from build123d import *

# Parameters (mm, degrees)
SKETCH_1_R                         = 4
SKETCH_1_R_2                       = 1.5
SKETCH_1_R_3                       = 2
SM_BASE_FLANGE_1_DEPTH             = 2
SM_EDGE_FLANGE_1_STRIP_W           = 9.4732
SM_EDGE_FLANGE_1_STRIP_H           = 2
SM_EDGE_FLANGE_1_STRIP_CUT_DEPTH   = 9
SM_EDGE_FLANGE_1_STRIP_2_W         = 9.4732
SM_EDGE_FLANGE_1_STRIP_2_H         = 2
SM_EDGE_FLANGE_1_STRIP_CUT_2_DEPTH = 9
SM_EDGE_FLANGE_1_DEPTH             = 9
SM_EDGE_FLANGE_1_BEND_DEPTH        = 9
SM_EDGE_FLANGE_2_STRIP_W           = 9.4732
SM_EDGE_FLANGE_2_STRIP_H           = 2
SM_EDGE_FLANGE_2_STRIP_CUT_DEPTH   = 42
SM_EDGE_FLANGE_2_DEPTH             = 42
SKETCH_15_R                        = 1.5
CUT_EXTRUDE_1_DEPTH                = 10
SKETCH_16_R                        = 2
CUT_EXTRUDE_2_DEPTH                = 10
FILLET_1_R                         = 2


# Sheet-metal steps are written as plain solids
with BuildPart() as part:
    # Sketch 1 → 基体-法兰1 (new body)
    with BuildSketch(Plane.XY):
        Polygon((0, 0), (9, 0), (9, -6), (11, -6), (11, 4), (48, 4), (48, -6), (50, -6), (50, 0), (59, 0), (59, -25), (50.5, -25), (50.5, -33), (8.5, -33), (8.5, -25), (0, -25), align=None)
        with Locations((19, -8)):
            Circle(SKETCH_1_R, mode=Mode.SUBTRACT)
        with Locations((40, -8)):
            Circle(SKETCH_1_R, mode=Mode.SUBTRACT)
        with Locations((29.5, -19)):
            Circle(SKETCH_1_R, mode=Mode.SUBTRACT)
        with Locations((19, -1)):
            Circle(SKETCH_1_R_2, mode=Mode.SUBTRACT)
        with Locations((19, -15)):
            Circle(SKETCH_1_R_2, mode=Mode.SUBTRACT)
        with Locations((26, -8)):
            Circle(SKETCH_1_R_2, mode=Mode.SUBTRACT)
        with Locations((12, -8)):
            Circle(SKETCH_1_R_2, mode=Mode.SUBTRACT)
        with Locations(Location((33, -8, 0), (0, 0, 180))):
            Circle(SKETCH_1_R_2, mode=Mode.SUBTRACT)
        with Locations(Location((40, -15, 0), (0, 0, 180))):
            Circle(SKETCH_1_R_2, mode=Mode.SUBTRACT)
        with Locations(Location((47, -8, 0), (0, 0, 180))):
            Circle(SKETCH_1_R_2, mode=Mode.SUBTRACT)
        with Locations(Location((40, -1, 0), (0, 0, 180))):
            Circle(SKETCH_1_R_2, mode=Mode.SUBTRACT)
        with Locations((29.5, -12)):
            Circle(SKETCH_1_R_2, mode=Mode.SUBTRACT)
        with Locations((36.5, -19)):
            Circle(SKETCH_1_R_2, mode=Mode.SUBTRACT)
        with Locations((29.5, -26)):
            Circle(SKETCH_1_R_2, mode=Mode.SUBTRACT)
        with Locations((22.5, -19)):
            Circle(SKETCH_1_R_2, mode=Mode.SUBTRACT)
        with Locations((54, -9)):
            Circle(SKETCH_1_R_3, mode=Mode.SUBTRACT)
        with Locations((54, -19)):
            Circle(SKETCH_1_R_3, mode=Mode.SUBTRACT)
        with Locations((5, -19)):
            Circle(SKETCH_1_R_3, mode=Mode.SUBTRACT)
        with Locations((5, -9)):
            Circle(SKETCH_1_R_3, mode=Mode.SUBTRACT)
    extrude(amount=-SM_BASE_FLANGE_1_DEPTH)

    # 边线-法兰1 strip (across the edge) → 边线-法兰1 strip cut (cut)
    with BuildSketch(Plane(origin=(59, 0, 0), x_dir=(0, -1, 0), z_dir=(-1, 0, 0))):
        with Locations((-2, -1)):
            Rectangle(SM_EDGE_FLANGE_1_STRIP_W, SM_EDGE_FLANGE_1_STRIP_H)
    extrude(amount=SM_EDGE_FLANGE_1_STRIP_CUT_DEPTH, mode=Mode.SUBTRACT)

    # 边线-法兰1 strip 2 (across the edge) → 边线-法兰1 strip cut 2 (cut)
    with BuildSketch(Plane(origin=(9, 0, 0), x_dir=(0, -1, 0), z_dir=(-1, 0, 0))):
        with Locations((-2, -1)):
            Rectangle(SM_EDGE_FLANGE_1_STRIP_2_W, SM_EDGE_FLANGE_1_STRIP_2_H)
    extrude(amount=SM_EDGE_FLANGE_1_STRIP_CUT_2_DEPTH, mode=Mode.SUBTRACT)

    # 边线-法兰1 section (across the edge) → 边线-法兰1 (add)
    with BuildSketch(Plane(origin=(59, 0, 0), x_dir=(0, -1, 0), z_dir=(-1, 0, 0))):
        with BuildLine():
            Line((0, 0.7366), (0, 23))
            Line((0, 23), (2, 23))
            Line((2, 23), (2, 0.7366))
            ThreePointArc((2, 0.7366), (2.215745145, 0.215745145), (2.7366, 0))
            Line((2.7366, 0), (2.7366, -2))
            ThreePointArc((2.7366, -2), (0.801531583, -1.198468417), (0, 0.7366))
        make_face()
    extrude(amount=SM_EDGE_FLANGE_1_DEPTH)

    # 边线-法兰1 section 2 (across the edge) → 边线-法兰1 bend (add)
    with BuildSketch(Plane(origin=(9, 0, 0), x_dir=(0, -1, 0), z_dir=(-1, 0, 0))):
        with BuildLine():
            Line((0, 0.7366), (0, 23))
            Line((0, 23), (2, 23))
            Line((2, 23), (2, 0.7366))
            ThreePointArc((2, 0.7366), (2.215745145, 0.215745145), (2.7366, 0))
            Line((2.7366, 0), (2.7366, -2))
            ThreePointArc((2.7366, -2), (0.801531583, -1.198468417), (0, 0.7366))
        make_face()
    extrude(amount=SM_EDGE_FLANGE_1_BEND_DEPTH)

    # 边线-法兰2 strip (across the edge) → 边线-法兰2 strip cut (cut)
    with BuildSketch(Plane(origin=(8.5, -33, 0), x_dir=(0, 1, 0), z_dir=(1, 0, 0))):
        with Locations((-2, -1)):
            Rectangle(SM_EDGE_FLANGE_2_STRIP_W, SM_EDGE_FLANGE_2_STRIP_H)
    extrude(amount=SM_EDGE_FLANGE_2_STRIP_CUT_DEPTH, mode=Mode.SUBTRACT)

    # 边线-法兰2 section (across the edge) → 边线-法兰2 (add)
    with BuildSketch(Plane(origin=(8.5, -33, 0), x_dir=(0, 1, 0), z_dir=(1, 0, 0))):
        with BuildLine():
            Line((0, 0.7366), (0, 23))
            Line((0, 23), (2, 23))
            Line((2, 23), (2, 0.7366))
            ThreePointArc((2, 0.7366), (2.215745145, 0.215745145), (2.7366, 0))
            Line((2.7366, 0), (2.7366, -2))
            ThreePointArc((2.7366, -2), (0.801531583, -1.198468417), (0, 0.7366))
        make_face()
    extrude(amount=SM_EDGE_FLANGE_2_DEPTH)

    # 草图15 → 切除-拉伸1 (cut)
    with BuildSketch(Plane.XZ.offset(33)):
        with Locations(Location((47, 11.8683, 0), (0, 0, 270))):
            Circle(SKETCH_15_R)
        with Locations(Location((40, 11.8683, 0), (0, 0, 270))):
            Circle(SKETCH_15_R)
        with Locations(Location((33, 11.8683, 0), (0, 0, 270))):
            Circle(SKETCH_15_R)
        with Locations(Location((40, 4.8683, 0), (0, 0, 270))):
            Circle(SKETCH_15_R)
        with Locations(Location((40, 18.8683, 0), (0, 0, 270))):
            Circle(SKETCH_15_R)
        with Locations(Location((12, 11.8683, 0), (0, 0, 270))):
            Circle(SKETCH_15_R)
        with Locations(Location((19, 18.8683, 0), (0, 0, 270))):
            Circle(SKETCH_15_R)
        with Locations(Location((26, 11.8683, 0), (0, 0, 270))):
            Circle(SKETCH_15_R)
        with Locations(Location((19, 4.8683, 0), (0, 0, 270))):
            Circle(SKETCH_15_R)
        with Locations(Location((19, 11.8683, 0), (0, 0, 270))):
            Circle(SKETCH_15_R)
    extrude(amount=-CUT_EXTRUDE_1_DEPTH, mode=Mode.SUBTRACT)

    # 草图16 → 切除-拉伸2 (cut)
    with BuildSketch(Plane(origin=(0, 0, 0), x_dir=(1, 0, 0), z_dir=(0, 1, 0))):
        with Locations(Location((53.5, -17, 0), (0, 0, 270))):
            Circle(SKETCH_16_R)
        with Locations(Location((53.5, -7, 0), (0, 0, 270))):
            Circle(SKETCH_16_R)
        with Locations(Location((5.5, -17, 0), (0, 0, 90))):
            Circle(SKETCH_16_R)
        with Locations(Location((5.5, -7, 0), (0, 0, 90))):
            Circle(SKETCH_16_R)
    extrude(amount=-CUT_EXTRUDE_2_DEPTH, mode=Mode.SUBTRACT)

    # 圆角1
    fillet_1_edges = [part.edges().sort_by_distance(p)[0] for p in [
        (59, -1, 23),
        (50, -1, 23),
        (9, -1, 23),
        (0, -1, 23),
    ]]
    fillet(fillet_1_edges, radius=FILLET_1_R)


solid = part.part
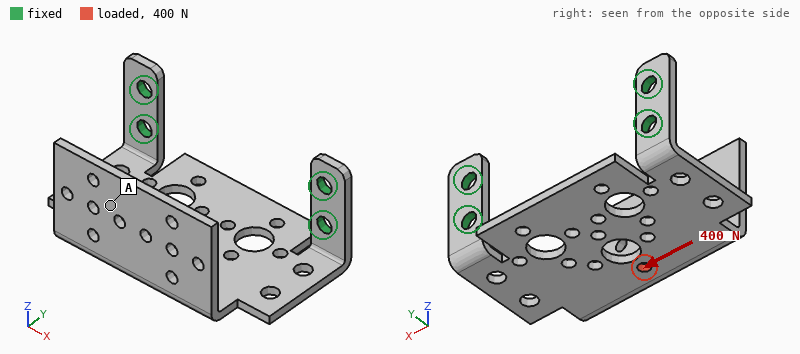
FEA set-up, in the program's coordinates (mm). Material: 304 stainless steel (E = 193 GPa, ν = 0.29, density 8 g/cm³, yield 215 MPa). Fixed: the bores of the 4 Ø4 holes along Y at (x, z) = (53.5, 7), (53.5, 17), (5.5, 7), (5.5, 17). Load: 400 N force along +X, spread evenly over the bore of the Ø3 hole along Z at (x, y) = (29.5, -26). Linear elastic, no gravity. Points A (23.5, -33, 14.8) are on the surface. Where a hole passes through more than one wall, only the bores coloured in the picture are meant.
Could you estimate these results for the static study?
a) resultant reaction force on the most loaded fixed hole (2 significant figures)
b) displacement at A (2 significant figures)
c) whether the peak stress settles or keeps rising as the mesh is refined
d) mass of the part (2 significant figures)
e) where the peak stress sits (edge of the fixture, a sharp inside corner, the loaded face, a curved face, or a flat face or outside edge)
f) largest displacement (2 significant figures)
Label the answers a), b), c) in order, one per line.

a) 310 N
b) 49 µm
c) keeps rising
d) 46 g
e) edge of the fixture
f) 66 µm
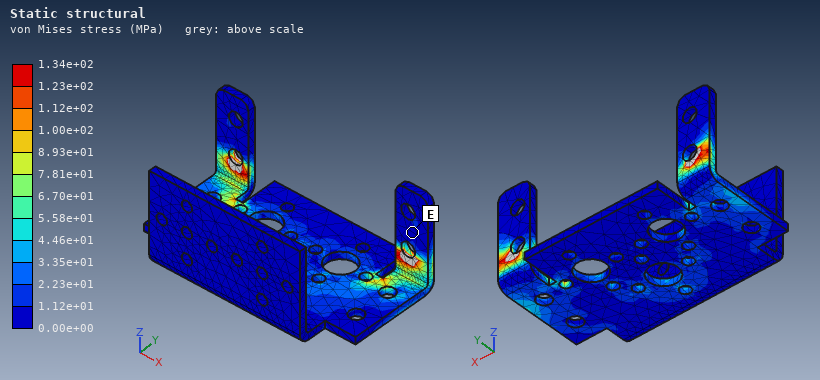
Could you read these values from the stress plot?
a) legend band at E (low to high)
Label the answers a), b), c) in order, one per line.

a) 0.00e+00 to 1.12e+01 MPa
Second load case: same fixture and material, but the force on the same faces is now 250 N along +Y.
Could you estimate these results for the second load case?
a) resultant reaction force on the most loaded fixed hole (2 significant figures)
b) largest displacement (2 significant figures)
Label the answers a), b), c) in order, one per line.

a) 130 N
b) 88 µm
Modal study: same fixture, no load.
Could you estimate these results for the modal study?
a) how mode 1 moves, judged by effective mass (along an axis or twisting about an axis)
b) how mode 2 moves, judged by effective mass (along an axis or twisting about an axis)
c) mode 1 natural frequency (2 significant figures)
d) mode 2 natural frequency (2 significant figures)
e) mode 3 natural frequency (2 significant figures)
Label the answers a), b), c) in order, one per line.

a) along Z
b) along X
c) 400 Hz
d) 1200 Hz
e) 1600 Hz
